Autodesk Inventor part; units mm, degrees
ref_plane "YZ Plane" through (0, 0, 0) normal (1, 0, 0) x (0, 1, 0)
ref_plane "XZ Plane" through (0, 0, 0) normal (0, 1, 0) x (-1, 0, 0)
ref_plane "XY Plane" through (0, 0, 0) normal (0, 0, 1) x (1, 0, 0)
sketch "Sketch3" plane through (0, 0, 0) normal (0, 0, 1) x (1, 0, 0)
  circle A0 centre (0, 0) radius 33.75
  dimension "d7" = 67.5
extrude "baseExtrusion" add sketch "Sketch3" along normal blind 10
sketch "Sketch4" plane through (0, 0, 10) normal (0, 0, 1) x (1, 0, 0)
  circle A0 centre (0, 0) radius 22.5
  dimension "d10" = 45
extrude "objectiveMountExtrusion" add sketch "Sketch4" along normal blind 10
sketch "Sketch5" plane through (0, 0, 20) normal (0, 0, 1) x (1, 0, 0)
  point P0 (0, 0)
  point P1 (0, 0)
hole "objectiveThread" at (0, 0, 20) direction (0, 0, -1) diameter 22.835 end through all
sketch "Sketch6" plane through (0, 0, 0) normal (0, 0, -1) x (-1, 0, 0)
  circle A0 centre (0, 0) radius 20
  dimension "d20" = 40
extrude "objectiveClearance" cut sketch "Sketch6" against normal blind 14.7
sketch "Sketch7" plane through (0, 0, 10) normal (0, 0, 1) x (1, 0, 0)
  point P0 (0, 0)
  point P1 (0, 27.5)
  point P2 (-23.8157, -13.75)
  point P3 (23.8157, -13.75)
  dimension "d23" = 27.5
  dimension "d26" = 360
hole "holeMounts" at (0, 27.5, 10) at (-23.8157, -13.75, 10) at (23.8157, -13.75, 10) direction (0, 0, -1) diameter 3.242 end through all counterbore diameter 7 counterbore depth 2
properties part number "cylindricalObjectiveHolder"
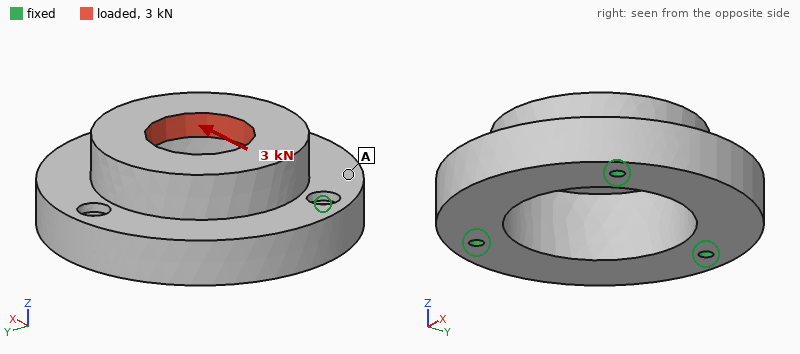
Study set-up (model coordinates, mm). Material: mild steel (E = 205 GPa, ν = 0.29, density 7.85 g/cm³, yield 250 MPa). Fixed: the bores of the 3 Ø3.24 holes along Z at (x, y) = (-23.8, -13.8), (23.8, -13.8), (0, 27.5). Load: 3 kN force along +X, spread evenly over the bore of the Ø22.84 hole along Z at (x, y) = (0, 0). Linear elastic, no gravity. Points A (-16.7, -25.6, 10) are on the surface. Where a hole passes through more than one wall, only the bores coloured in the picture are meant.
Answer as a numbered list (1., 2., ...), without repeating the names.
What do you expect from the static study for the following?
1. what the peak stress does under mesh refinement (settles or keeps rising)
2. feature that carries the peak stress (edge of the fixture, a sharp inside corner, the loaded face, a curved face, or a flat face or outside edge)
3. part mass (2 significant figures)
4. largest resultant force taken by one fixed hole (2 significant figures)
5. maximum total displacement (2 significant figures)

1. keeps rising
2. edge of the fixture
3. 240 g
4. 1.2 kN
5. 4.8 µm
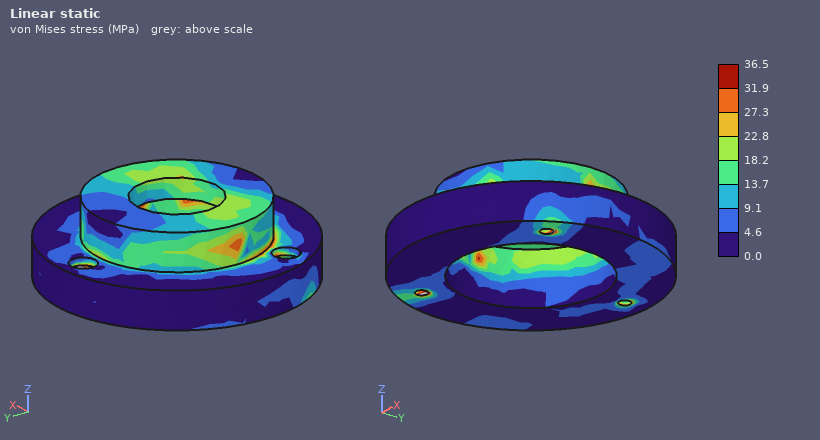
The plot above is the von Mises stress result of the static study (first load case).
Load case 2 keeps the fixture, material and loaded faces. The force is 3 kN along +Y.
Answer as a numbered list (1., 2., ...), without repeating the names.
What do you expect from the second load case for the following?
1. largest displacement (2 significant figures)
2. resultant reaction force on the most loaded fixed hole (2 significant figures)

1. 5.2 µm
2. 1.2 kN
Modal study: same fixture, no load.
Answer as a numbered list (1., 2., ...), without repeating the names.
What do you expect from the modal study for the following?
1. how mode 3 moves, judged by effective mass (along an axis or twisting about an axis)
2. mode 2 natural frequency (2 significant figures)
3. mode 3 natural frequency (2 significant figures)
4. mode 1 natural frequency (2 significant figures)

1. along Z
2. 11 kHz
3. 14 kHz
4. 11 kHz
